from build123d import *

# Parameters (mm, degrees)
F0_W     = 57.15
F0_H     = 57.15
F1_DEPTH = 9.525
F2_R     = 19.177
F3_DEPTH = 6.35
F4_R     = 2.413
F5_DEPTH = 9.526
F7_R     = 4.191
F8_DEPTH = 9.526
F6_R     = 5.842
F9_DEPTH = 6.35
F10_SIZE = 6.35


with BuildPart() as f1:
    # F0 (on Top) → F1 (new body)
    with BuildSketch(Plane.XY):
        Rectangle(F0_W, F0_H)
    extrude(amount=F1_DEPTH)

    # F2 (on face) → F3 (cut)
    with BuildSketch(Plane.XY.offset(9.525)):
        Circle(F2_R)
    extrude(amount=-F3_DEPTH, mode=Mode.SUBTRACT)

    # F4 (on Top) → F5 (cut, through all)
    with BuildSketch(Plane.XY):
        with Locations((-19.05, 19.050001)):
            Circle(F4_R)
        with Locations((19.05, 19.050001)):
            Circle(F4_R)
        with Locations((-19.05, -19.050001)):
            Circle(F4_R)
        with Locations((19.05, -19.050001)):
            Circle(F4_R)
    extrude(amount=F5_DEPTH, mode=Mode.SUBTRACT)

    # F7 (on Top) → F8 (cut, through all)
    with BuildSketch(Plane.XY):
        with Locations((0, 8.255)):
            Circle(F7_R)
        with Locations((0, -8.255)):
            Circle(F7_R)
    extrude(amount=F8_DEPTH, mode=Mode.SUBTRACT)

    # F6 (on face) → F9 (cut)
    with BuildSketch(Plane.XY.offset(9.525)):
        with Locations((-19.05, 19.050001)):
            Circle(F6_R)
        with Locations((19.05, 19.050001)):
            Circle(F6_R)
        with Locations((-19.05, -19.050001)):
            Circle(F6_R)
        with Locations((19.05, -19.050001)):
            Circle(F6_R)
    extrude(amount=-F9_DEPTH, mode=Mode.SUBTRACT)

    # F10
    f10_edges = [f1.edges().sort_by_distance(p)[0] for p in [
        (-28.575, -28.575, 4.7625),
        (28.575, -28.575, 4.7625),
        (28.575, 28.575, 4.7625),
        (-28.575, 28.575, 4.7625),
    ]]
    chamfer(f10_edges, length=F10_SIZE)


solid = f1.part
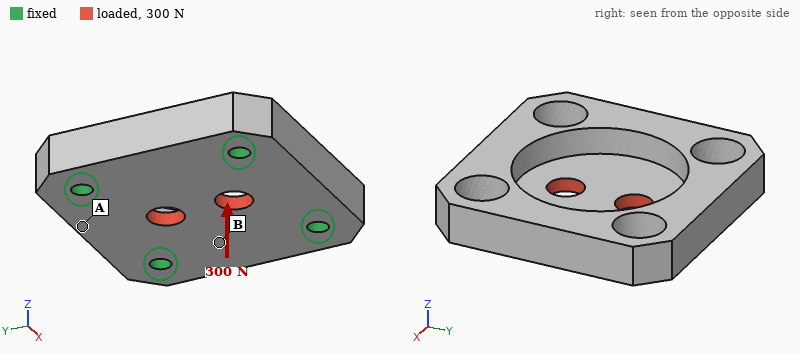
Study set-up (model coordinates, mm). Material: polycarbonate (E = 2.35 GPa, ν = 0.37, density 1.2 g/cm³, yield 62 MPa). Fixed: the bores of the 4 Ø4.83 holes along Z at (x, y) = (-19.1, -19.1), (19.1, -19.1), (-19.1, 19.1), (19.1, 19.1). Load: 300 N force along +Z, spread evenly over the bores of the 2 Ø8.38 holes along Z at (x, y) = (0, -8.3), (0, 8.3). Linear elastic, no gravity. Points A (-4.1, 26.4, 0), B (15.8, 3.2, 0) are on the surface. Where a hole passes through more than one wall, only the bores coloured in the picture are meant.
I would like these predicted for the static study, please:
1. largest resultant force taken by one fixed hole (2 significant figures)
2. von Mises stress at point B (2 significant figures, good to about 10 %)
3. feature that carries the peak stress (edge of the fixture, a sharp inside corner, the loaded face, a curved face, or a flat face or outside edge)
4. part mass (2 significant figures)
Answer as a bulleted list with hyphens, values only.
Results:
- 91 N
- 6.3 MPa
- the loaded face
- 24 g
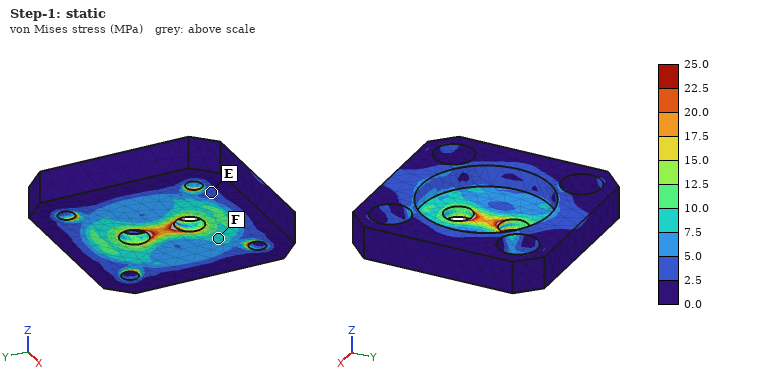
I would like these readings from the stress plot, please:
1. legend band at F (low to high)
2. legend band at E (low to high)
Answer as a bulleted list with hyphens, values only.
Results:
- 7.5 to 10.0 MPa
- 2.5 to 5.0 MPa
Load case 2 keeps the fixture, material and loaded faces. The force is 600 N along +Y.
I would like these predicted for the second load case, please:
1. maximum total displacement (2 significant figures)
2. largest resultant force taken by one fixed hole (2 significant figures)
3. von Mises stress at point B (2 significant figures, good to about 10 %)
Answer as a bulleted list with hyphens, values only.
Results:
- 51 µm
- 160 N
- 1.6 MPa
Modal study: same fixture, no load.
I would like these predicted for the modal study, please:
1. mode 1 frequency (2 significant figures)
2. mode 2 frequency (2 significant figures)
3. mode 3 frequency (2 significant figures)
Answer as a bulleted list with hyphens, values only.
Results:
- 3500 Hz
- 3600 Hz
- 4400 Hz
